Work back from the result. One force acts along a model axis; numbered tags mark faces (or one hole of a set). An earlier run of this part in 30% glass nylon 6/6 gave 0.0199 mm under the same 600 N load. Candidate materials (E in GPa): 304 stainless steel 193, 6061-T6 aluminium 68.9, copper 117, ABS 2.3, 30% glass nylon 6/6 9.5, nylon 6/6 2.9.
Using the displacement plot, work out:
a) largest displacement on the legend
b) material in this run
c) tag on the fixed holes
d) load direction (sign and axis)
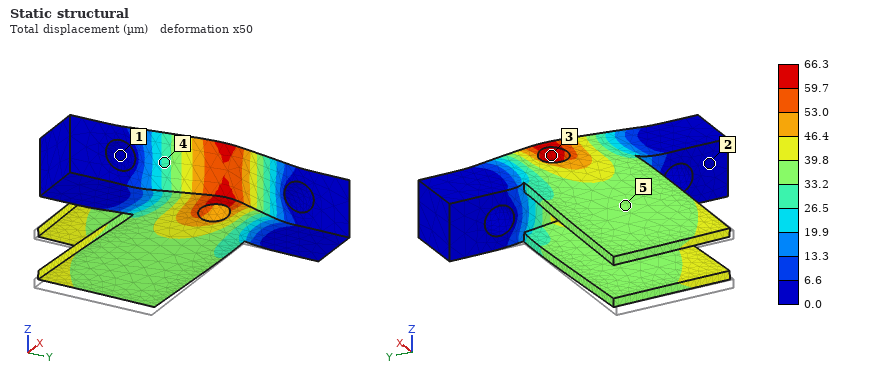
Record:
66.3 µm
nylon 6/6
1
+X
